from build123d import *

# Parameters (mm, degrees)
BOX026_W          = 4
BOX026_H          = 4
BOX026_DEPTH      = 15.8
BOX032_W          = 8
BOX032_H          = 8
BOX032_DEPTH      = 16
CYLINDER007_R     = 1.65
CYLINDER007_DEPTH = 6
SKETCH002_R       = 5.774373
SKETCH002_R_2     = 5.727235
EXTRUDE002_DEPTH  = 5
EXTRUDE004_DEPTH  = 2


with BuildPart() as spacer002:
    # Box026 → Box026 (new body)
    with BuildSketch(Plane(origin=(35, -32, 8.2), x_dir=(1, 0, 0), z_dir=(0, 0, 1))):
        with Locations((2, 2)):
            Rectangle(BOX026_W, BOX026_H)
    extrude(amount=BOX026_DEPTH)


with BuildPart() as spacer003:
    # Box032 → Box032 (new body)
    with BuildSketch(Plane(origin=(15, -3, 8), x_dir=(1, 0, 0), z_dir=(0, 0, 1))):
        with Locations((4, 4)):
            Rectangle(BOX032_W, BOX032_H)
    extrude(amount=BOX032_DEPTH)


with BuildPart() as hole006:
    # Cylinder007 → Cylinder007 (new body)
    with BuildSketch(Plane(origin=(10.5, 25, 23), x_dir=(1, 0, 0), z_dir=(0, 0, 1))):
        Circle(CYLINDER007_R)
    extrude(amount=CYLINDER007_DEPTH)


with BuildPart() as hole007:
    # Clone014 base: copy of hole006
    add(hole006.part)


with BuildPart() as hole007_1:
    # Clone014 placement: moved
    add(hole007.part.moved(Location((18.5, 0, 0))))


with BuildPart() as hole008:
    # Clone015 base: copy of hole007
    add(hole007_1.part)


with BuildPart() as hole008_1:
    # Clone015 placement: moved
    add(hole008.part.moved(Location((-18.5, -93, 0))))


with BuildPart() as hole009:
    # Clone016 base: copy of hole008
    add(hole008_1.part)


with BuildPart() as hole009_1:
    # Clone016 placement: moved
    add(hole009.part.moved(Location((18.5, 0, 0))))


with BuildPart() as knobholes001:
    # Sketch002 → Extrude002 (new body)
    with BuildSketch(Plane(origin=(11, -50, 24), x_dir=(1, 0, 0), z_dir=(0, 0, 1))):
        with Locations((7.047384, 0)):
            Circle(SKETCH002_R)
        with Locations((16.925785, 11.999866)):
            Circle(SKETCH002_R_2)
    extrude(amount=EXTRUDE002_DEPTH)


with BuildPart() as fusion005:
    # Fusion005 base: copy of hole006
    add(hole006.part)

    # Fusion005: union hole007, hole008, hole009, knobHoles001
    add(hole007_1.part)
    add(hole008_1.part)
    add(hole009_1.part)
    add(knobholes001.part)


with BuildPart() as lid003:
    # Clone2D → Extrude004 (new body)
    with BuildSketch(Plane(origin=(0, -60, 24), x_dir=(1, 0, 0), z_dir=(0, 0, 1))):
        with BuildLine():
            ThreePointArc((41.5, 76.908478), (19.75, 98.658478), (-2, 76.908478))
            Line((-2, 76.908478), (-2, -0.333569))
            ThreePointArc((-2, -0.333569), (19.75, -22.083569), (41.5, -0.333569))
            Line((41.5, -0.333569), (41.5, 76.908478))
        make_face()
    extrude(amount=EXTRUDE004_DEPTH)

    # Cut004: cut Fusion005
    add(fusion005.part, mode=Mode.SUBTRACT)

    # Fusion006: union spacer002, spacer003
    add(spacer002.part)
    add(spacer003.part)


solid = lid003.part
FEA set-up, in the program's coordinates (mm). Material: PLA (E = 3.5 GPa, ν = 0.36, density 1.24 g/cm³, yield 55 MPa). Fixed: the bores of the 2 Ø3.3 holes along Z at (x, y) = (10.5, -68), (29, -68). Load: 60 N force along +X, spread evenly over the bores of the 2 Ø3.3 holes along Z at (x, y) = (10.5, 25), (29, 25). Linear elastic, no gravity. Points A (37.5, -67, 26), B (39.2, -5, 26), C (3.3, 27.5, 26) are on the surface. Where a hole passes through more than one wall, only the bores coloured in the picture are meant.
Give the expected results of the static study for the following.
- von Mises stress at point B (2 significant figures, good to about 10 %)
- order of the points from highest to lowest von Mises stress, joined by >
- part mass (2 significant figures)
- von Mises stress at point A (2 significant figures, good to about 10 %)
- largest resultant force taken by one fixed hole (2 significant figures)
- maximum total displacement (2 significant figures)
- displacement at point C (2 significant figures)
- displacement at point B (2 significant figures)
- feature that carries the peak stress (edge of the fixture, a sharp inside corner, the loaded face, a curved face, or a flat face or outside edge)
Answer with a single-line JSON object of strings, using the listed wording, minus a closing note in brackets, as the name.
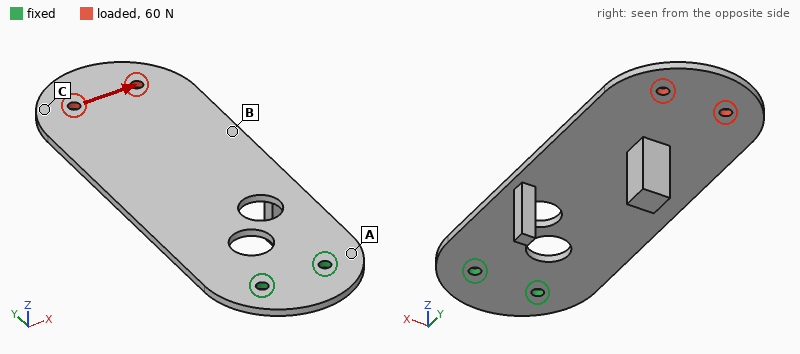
{"von Mises stress at point B": "2.7 MPa", "order of the points from highest to lowest von Mises stress, joined by >": "A > B > C", "part mass": "13 g", "von Mises stress at point A": "5.3 MPa", "largest resultant force taken by one fixed hole": "270 N", "maximum total displacement": "0.78 mm", "displacement at point C": "0.70 mm", "displacement at point B": "0.44 mm", "feature that carries the peak stress": "edge of the fixture"}
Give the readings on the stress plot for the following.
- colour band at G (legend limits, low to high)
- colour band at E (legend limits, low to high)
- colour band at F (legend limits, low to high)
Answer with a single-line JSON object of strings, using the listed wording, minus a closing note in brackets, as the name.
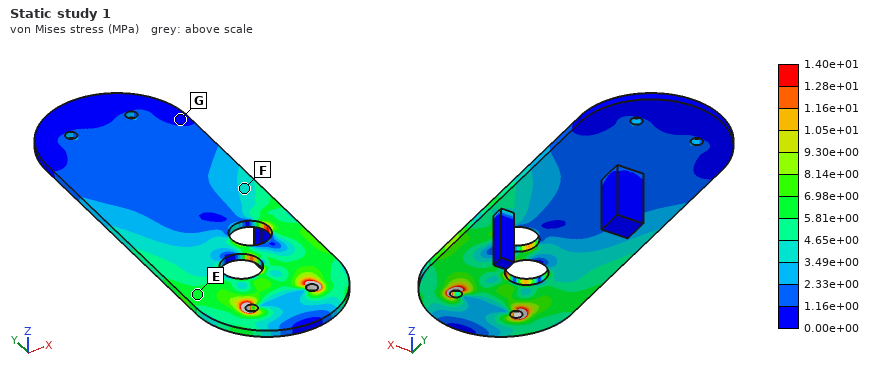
{"colour band at G": "0.00e+00 to 1.16e+00 MPa", "colour band at E": "5.81e+00 to 6.98e+00 MPa", "colour band at F": "3.49e+00 to 4.65e+00 MPa"}
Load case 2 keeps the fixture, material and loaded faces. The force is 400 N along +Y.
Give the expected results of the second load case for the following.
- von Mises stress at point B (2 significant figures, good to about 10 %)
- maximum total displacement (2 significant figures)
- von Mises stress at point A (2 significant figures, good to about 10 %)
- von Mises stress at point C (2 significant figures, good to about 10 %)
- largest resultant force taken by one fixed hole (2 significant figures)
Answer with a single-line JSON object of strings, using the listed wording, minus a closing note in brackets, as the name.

{"von Mises stress at point B": "5.0 MPa", "maximum total displacement": "0.20 mm", "von Mises stress at point A": "3.6 MPa", "von Mises stress at point C": "2.5 MPa", "largest resultant force taken by one fixed hole": "200 N"}
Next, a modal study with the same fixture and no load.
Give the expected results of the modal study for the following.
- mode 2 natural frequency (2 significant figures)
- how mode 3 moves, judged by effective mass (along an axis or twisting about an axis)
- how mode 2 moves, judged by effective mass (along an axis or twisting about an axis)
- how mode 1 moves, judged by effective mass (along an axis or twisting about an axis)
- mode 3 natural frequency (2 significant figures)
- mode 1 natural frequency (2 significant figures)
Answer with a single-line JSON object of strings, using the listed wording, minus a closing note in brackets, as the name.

{"mode 2 natural frequency": "230 Hz", "how mode 3 moves, judged by effective mass": "along Z", "how mode 2 moves, judged by effective mass": "twisting about Y", "how mode 1 moves, judged by effective mass": "along Z", "mode 3 natural frequency": "310 Hz", "mode 1 natural frequency": "45 Hz"}
